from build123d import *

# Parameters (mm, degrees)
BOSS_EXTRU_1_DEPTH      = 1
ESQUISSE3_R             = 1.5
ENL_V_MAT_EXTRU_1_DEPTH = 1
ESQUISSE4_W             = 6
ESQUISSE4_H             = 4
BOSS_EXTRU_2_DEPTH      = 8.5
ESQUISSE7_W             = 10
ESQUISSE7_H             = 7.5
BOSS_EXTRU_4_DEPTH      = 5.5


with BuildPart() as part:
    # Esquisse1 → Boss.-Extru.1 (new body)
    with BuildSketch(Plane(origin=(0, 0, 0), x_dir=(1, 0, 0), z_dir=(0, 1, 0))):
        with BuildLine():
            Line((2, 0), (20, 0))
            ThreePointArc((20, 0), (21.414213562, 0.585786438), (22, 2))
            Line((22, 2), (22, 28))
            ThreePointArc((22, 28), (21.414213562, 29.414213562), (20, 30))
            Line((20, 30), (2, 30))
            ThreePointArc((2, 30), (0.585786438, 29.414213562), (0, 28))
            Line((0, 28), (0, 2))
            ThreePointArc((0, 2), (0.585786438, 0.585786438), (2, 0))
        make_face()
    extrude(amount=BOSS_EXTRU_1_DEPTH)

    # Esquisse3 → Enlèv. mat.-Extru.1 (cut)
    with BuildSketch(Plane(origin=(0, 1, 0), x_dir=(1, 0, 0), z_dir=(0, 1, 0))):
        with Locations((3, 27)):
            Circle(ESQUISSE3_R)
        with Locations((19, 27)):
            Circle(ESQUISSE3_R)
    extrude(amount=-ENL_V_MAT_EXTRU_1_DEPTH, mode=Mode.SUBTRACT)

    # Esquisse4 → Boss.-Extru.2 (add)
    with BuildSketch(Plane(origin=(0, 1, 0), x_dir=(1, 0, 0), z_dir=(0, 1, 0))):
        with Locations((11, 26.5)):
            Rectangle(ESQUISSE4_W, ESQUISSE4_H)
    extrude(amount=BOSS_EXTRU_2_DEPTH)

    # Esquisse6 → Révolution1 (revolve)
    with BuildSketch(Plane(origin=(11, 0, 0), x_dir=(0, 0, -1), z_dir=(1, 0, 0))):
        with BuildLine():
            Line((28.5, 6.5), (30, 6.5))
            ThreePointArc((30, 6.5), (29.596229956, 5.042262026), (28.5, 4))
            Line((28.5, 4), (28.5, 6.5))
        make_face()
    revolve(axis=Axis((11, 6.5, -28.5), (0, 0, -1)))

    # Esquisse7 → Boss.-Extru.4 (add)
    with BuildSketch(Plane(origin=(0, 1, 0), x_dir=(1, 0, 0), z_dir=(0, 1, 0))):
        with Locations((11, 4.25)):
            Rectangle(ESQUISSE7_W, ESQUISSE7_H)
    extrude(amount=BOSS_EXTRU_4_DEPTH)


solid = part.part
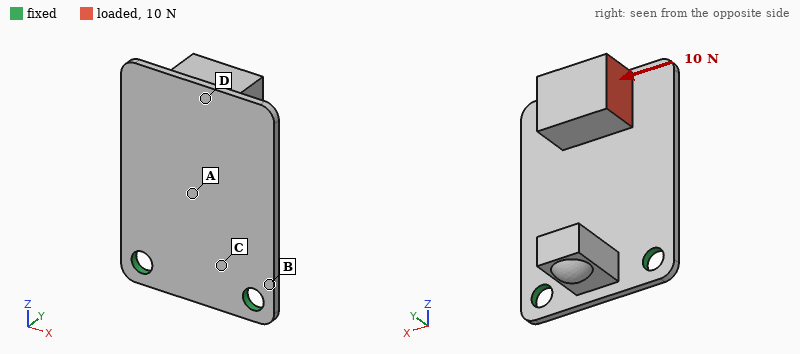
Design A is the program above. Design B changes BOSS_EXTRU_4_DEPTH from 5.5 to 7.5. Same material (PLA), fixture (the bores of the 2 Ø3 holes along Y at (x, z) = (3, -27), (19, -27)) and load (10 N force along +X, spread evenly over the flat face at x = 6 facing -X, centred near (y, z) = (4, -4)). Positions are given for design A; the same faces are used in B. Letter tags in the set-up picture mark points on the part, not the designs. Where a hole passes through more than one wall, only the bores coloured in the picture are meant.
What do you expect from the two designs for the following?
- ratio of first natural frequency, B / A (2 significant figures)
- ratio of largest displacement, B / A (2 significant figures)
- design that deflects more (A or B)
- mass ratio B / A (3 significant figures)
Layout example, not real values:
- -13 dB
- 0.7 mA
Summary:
- 0.89
- 1.3
- B
- 1.12
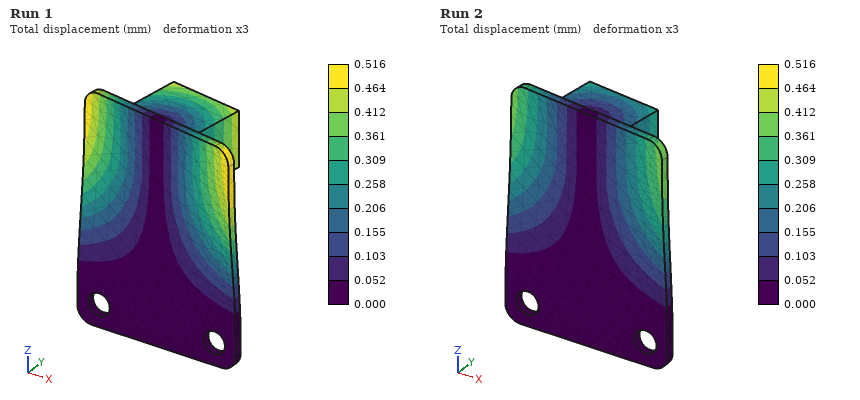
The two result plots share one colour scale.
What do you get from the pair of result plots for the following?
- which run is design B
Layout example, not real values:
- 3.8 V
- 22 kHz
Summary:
- Run 1
